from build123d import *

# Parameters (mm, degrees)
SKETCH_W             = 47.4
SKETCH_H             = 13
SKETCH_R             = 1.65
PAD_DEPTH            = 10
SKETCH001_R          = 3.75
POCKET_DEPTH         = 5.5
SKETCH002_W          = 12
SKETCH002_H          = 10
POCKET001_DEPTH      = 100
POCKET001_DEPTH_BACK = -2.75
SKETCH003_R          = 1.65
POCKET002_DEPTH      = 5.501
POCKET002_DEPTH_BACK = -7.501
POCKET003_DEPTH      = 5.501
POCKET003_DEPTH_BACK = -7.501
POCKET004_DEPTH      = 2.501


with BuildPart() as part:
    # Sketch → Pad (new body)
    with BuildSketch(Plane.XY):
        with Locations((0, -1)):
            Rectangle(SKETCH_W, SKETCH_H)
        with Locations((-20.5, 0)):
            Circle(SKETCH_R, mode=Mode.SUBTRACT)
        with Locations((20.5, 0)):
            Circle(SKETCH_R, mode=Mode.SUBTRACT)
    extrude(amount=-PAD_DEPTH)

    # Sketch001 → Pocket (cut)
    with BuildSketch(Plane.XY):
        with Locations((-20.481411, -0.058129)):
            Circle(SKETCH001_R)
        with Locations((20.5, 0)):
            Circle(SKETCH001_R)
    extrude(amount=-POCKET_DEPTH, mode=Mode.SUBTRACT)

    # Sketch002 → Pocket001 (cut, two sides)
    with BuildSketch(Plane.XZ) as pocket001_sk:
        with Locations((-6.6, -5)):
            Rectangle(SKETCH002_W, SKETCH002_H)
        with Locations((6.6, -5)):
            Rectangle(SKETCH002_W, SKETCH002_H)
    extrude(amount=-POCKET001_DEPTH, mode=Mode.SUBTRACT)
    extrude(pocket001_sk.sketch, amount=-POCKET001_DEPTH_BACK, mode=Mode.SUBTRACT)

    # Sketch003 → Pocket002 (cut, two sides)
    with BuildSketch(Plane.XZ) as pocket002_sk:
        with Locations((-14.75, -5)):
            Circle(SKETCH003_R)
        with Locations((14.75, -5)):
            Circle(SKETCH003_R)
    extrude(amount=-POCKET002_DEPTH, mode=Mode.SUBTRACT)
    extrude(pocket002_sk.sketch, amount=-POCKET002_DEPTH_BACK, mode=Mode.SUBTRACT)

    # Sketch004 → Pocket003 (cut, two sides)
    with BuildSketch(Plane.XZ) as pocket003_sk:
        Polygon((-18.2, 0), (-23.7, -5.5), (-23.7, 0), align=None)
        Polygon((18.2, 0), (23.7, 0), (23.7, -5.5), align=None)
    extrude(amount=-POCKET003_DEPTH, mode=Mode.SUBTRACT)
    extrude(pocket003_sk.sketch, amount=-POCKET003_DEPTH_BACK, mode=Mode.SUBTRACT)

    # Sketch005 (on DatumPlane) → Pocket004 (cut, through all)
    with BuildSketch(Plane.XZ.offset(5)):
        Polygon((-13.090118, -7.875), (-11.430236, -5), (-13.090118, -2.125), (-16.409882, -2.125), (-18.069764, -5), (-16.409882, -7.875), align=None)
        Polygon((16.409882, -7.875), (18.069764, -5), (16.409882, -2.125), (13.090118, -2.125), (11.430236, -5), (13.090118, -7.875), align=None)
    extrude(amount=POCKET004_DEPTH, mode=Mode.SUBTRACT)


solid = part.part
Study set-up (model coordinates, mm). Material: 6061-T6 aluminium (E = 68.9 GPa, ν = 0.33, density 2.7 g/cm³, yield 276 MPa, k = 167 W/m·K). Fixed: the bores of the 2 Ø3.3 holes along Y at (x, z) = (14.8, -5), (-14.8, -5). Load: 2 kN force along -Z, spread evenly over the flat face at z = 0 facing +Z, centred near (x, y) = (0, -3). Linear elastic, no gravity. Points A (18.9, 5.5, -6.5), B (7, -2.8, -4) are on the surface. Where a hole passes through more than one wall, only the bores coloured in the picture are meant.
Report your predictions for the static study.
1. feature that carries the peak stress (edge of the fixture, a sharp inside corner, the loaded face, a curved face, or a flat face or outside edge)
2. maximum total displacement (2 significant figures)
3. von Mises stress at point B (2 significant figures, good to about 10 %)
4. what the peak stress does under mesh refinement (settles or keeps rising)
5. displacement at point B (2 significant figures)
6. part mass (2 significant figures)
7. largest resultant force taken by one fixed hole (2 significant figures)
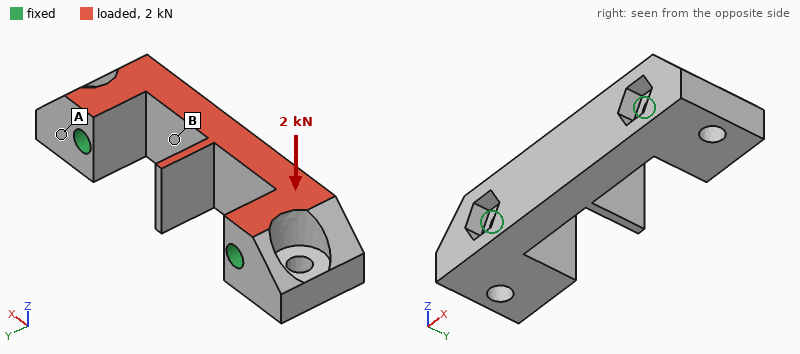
edge of the fixture
15 µm
22 MPa
keeps rising
7.2 µm
8.4 g
1.0 kN
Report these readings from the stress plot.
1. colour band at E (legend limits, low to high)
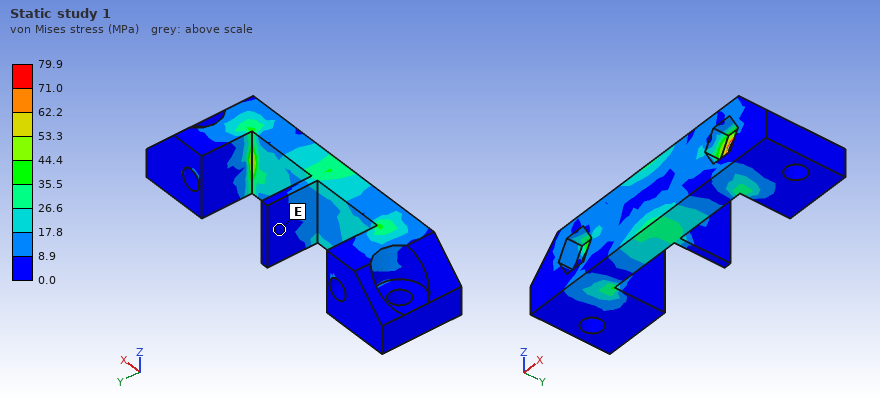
0.0 to 8.9 MPa
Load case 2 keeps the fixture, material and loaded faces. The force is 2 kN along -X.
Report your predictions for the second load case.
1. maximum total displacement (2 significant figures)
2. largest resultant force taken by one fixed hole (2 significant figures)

0.10 mm
1.0 kN
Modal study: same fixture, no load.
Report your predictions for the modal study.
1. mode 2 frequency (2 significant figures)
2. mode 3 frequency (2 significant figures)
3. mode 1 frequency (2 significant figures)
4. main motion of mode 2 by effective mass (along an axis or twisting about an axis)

22 kHz
25 kHz
14 kHz
along Y
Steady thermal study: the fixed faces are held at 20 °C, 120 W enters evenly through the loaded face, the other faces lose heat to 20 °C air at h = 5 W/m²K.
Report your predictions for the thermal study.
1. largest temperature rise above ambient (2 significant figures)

60 K
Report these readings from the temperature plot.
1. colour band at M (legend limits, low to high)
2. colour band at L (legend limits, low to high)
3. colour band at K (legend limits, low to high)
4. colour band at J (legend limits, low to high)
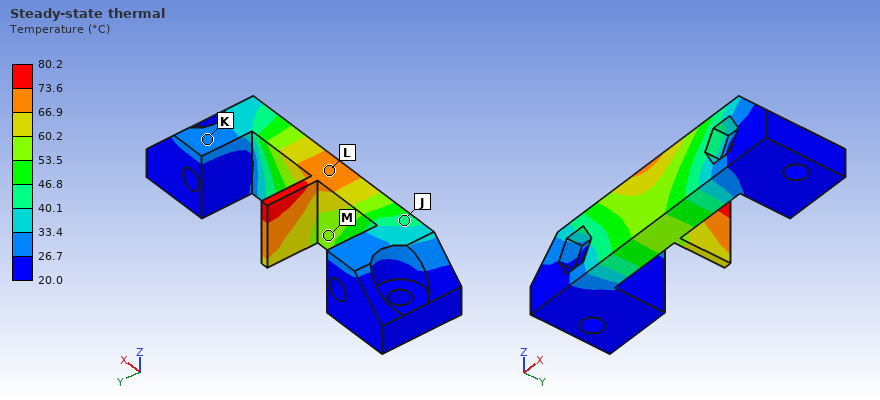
53.5 to 60.2 °C
66.9 to 73.6 °C
26.7 to 33.4 °C
40.1 to 46.8 °C
